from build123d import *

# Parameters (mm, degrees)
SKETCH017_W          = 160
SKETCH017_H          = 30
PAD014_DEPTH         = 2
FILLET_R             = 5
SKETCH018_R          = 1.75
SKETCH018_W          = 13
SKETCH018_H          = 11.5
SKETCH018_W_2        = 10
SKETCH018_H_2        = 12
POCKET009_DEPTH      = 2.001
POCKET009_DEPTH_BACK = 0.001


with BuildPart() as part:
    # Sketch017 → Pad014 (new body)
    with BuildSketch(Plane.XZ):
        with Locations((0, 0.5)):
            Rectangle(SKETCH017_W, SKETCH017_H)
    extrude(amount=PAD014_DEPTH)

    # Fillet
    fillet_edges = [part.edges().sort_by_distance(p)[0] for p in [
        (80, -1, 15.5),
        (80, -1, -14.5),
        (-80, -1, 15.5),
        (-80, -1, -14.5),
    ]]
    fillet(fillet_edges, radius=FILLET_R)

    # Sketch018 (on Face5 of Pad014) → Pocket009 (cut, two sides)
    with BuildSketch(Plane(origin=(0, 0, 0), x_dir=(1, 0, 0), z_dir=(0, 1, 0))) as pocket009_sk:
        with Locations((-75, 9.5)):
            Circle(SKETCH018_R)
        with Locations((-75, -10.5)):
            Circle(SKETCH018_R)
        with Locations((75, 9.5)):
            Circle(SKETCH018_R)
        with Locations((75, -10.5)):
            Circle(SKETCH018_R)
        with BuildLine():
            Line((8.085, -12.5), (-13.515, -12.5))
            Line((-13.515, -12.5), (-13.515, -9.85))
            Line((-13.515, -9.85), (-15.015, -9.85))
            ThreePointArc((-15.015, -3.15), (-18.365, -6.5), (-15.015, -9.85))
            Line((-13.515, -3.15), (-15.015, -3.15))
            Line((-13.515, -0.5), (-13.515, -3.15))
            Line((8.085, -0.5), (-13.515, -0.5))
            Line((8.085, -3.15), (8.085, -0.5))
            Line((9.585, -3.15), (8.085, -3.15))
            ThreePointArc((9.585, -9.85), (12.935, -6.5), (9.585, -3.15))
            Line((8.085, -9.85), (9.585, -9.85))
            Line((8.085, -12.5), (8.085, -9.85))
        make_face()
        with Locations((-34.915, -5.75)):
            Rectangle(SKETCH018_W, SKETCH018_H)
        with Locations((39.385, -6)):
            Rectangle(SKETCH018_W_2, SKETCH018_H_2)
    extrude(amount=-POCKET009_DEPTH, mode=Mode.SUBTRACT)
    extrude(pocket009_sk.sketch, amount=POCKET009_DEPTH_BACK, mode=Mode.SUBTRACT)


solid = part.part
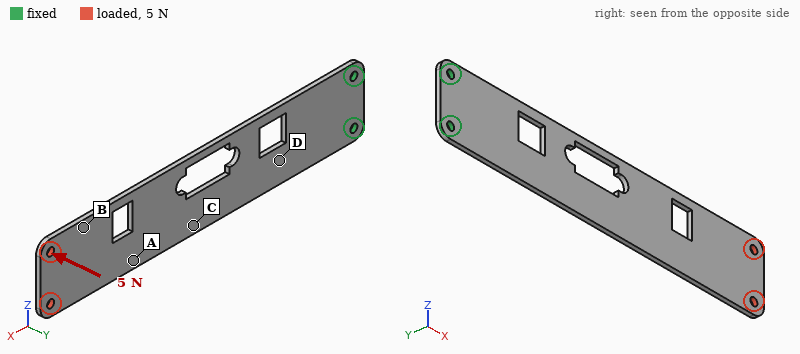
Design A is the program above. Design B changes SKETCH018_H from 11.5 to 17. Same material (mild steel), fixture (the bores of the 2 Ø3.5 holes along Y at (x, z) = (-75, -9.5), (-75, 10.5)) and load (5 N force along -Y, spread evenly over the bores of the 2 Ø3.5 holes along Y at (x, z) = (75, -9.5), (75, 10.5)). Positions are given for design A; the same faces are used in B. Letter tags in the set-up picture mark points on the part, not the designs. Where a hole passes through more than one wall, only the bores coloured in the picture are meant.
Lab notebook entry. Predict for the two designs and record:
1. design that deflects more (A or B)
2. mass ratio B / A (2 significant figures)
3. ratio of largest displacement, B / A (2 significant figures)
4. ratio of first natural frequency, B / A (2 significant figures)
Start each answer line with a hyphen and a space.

- B
- 0.98
- 1.1
- 0.93
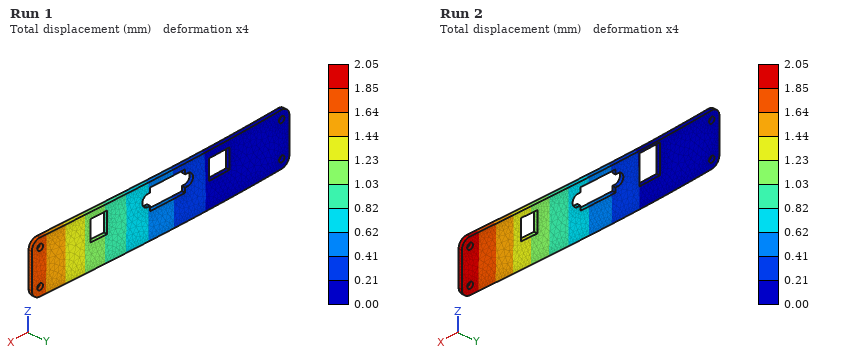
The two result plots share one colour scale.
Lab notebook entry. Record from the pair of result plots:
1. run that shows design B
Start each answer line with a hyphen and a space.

- Run 2
